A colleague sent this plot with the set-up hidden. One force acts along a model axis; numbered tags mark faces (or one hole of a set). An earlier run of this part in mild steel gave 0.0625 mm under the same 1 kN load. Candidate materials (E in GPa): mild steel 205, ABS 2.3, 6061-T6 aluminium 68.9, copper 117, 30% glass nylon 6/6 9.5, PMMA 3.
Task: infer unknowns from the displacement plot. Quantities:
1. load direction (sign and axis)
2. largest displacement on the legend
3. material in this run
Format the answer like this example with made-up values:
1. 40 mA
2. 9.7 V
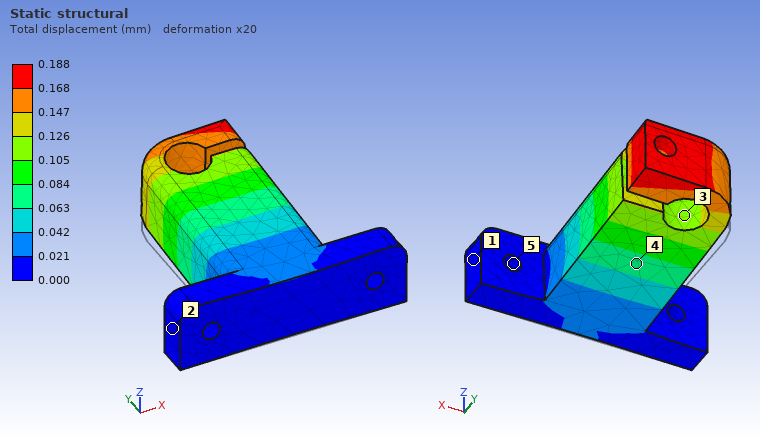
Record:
1. +Z
2. 0.188 mm
3. 6061-T6 aluminium
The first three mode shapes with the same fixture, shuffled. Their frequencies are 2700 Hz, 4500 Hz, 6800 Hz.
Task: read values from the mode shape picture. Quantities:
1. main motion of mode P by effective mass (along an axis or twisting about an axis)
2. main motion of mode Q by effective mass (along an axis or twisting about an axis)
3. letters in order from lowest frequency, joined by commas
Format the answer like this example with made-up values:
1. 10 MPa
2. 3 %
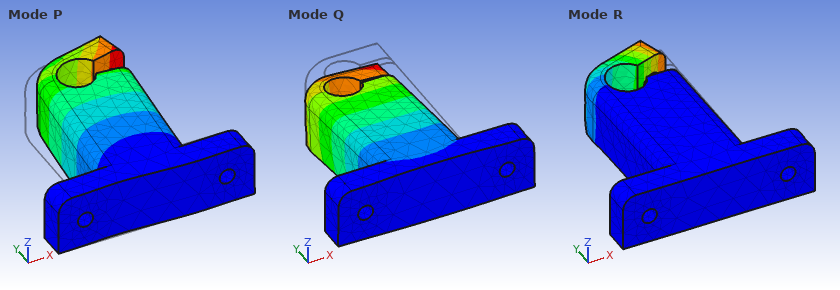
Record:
1. along X
2. along Z
3. Q, R, P
